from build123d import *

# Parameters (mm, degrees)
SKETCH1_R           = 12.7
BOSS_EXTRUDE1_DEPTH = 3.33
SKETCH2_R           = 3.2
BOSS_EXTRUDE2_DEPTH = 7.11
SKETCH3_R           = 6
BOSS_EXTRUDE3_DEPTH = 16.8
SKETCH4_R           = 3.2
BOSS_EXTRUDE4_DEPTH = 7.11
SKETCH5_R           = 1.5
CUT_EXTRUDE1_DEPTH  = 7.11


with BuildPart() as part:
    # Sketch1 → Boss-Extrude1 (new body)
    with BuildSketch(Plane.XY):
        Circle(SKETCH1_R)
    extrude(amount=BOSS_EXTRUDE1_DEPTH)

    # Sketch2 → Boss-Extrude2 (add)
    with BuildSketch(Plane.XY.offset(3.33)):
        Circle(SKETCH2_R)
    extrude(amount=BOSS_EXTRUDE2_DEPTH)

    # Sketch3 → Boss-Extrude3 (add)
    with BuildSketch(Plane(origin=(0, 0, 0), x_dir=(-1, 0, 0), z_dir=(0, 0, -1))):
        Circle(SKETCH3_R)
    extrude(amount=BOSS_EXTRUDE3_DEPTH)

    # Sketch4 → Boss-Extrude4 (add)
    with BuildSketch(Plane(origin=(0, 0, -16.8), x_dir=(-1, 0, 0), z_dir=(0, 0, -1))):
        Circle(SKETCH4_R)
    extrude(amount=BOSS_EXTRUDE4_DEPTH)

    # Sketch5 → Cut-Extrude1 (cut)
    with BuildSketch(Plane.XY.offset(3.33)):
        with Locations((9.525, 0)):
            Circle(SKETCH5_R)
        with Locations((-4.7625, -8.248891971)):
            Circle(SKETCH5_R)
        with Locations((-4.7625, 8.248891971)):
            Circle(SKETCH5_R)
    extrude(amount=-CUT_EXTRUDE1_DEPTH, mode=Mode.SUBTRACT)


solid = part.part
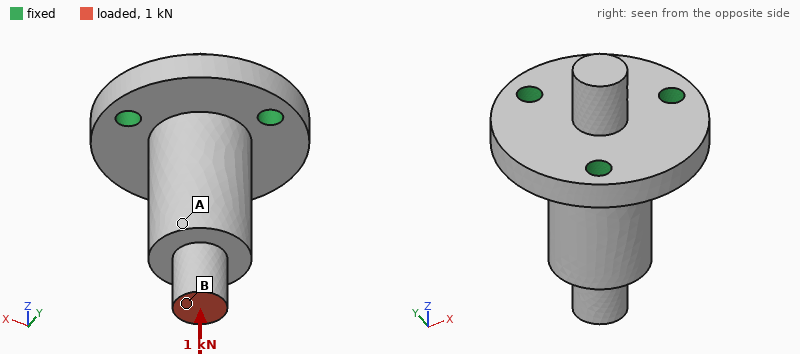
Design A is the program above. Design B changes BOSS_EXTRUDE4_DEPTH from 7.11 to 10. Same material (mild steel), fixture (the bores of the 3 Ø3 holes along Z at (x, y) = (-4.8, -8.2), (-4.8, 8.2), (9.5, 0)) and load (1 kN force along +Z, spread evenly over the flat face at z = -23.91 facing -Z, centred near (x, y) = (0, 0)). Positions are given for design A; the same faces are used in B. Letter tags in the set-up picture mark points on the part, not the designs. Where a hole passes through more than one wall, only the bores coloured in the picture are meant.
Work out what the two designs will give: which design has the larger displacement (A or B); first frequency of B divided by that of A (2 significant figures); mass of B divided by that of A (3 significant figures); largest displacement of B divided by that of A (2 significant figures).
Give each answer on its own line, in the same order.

B
0.90
1.02
1.1
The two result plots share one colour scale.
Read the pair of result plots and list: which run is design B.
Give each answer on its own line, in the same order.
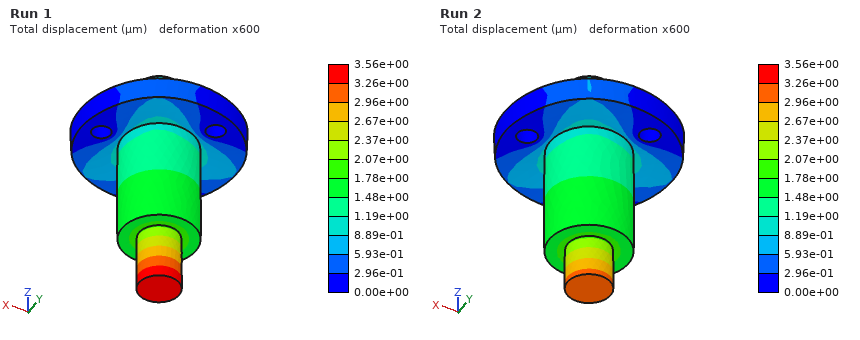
Run 1
